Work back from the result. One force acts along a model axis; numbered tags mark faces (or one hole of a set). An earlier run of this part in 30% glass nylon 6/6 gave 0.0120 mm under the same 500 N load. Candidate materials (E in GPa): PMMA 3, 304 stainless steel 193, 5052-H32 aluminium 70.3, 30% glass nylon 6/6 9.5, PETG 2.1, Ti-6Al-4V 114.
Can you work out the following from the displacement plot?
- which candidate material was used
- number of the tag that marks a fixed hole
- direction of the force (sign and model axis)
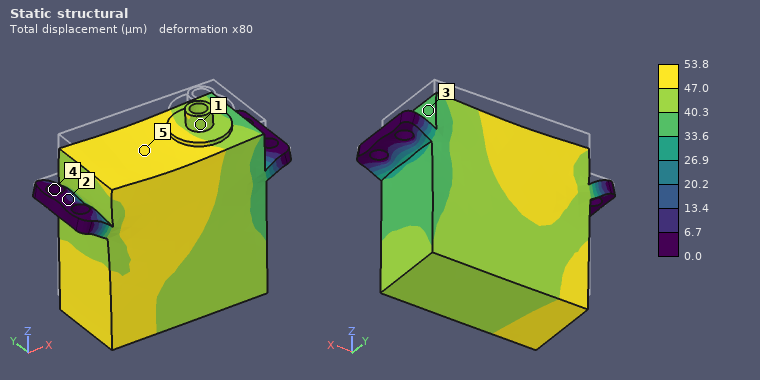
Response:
PETG
4
-Z
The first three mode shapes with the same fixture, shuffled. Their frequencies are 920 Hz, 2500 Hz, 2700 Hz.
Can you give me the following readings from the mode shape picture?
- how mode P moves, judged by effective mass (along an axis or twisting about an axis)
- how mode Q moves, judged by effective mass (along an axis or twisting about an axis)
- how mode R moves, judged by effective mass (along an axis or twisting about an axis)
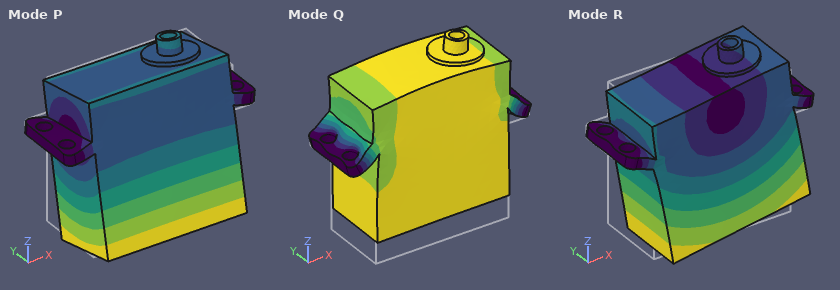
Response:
along Y
along Z
along X
